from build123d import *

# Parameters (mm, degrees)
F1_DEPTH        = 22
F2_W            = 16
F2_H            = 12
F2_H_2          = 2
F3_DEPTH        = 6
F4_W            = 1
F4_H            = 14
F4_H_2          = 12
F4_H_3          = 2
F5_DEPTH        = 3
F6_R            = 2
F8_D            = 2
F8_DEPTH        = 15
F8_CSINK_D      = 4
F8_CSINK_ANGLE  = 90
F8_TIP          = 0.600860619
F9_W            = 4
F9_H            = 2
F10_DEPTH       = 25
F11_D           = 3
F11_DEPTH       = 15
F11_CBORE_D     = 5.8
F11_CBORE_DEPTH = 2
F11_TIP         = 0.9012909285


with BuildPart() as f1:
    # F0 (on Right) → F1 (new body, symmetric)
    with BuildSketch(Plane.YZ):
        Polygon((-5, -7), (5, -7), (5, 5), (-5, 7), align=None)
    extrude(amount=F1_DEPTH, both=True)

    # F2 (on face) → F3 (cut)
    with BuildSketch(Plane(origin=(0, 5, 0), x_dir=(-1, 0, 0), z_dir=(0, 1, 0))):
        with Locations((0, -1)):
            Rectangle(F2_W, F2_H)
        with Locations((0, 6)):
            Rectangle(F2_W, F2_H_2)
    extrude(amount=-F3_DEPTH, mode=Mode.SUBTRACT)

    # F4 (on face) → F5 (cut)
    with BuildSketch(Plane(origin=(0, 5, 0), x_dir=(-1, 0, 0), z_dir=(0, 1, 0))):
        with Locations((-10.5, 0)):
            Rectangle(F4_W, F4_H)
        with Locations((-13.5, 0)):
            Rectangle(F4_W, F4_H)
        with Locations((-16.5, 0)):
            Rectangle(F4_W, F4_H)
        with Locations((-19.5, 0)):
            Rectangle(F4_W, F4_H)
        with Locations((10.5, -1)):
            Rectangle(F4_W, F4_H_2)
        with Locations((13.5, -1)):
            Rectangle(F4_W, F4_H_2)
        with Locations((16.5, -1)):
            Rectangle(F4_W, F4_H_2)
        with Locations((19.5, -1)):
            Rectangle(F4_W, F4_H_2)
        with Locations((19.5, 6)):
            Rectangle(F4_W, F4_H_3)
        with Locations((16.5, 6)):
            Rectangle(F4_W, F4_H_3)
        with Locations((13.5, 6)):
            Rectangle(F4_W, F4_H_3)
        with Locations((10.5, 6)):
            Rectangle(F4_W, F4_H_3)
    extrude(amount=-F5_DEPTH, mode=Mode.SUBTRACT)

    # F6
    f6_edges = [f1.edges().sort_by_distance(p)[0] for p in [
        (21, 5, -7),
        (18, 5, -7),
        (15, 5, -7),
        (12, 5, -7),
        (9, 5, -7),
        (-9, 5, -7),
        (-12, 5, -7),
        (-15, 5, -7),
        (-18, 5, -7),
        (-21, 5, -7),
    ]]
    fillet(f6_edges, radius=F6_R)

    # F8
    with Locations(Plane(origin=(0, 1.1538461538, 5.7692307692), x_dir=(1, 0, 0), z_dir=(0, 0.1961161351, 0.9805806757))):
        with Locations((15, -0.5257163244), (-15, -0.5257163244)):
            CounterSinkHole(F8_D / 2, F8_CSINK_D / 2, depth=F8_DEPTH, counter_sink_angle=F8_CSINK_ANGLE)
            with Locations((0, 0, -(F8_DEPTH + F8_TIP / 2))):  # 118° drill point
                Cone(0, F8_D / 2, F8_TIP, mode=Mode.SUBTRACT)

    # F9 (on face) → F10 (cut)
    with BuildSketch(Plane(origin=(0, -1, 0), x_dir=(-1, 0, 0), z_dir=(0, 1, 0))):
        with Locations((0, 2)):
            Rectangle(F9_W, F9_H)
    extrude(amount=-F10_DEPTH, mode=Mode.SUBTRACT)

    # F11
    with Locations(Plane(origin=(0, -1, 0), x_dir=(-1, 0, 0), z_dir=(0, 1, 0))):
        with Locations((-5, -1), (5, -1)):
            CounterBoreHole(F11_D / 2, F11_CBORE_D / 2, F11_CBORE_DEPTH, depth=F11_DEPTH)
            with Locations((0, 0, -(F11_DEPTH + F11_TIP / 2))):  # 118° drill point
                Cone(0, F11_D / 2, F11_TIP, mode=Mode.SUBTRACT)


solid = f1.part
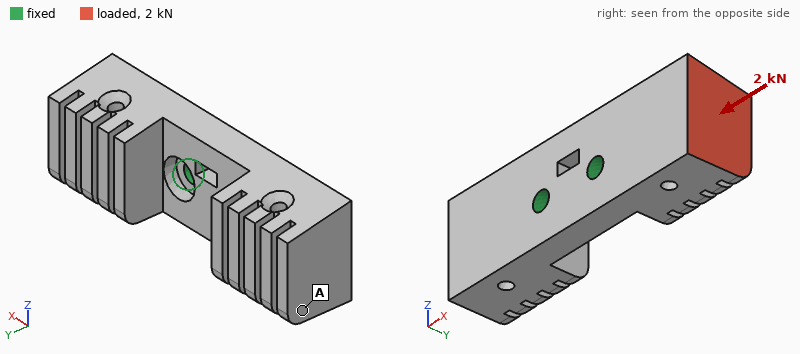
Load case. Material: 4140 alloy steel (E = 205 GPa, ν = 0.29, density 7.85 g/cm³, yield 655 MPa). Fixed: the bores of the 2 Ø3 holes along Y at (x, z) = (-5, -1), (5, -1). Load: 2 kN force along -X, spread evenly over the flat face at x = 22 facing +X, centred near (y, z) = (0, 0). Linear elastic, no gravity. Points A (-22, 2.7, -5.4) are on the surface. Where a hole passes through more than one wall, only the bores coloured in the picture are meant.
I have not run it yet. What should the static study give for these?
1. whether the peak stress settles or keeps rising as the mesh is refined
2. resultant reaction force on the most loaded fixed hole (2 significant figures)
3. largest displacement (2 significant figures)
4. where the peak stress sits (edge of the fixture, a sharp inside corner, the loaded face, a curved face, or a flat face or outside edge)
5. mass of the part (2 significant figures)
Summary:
keeps rising
1.2 kN
73 µm
edge of the fixture
31 g
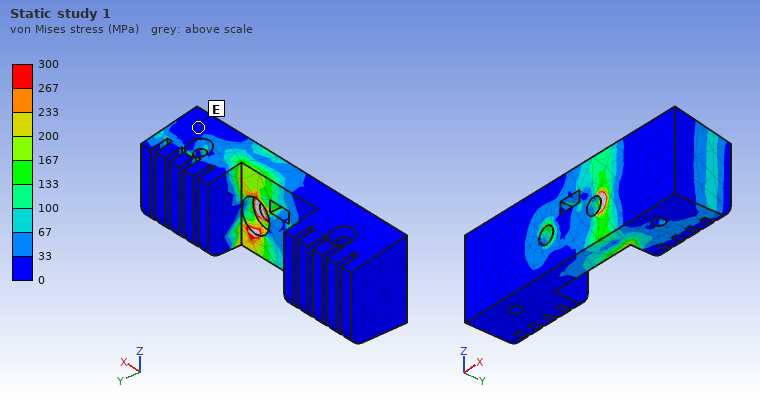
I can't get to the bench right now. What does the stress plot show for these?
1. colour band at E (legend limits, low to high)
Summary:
0 to 33 MPa
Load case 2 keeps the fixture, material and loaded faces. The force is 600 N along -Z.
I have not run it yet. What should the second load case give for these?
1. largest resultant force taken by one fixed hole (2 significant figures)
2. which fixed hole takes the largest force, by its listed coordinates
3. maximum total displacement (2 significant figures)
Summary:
1.2 kN
(5, -1)
27 µm
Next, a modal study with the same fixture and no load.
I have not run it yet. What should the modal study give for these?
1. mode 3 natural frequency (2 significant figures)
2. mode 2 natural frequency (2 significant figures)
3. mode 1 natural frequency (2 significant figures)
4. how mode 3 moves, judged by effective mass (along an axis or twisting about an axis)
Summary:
9400 Hz
5700 Hz
5700 Hz
along Z
